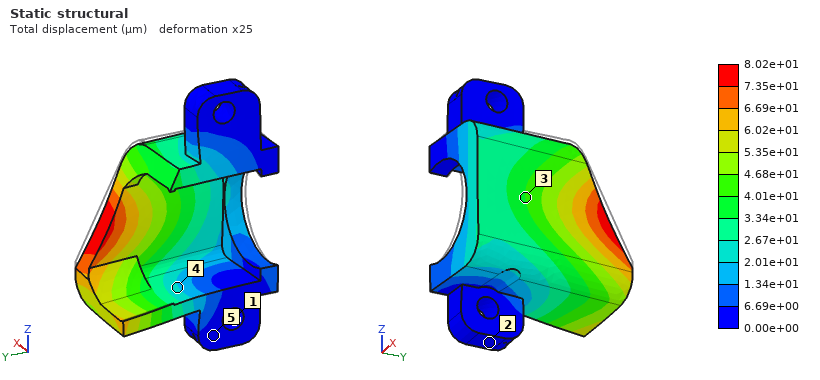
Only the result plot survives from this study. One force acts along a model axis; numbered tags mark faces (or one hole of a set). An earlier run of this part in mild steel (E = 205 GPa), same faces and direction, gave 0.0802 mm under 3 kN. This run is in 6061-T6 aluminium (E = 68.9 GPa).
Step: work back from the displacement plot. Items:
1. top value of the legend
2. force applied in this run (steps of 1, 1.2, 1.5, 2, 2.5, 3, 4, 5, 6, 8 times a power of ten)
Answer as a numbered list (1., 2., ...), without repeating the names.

1. 8.02e+01 µm
2. 1 kN
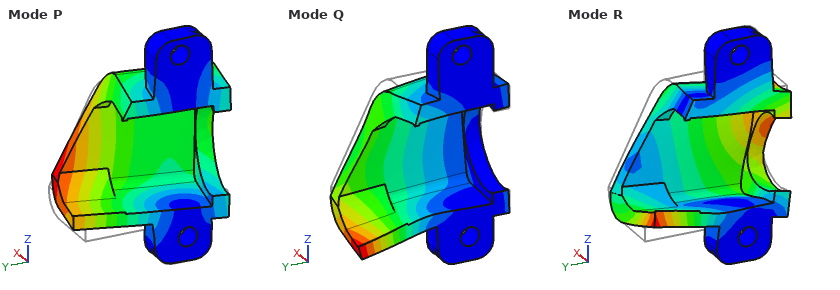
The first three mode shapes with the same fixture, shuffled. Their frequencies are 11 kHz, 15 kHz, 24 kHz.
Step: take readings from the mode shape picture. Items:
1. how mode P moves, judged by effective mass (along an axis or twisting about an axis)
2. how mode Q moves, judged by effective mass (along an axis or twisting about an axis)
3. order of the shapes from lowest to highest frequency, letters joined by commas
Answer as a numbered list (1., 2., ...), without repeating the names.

1. along Y
2. along Z
3. P, Q, R
